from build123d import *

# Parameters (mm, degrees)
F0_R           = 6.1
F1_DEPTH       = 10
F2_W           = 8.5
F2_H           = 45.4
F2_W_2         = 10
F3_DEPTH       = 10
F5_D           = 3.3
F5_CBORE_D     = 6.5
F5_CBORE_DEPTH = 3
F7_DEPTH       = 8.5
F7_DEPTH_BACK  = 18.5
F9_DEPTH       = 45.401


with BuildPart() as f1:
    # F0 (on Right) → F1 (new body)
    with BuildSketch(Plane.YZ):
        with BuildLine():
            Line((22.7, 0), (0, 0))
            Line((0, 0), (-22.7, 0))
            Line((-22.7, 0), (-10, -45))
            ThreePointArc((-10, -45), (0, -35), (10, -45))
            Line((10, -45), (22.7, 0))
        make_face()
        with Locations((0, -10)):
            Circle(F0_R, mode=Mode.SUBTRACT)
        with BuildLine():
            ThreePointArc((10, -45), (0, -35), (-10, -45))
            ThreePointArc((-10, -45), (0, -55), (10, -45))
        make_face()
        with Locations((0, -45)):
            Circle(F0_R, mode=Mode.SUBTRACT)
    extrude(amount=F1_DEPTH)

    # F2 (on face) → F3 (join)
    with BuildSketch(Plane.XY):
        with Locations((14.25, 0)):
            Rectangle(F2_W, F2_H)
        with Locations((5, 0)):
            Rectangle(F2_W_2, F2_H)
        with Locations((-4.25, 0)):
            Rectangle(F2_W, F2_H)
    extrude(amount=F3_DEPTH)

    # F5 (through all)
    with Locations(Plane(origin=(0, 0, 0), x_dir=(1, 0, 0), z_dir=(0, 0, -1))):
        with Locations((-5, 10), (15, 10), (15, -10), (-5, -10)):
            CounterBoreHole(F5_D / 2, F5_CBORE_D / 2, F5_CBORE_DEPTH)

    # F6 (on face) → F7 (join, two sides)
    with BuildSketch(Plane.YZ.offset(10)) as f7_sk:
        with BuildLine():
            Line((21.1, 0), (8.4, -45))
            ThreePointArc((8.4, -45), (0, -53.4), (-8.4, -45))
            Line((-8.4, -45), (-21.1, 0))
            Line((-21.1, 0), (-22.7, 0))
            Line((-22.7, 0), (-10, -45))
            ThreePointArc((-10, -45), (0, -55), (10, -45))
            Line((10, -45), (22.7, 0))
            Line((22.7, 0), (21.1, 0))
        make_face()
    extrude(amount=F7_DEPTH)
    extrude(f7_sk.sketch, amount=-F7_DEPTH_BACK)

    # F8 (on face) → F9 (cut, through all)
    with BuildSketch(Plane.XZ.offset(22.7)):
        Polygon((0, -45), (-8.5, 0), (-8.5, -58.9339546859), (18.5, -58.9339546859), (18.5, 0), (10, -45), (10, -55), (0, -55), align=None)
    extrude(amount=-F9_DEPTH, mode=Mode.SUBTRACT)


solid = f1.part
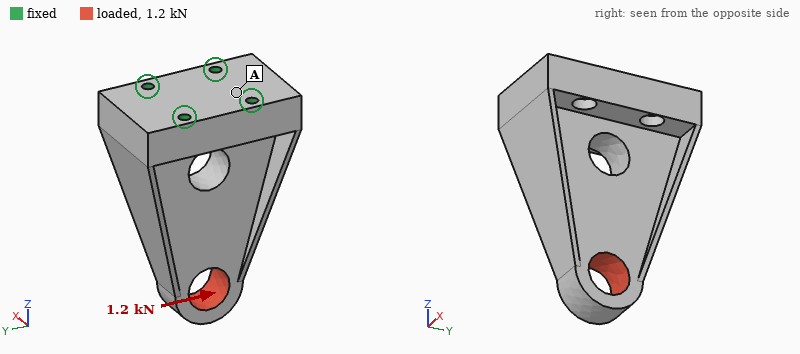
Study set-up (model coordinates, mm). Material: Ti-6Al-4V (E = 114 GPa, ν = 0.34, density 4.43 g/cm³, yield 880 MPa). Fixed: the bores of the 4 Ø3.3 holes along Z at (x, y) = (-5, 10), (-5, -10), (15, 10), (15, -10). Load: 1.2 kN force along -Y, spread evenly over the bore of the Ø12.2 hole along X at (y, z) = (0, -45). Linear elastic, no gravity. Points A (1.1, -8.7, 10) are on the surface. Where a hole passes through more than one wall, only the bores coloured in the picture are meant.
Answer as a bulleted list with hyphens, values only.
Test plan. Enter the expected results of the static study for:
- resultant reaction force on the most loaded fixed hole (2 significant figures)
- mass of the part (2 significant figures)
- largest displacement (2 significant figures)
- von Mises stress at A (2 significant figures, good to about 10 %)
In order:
- 1.3 kN
- 120 g
- 34 µm
- 12 MPa
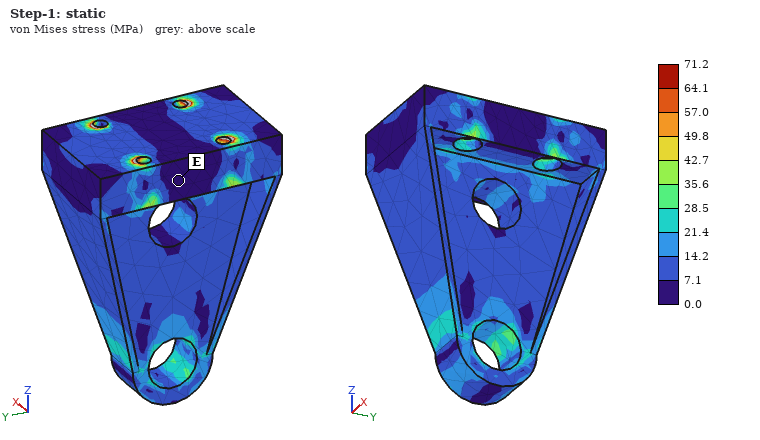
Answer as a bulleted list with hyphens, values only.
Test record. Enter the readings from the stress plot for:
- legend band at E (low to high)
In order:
- 0.0 to 7.1 MPa
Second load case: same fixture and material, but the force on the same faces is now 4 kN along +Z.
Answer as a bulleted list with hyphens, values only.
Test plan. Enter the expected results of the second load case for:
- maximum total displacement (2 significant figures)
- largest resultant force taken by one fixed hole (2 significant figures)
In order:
- 13 µm
- 1.0 kN
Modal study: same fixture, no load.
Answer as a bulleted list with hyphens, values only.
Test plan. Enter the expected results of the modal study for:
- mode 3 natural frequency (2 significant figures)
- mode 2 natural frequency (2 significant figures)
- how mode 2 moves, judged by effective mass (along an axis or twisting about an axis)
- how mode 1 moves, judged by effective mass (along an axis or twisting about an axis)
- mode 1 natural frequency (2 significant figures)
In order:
- 12 kHz
- 7000 Hz
- along Y
- along X
- 4100 Hz
